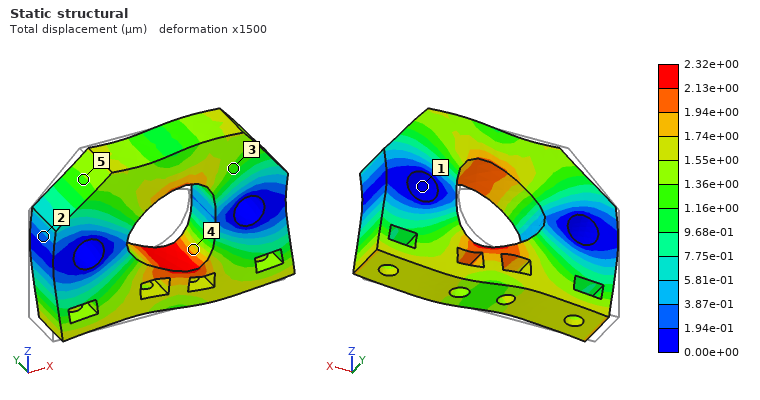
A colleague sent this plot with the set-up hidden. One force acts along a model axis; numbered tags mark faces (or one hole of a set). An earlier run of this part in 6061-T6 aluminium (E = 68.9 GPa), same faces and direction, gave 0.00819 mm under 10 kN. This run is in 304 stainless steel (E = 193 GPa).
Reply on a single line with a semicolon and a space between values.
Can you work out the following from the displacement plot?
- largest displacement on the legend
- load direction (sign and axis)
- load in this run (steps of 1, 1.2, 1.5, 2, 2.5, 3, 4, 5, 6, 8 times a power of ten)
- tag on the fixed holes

2.32e+00 µm; +X; 8 kN; 1
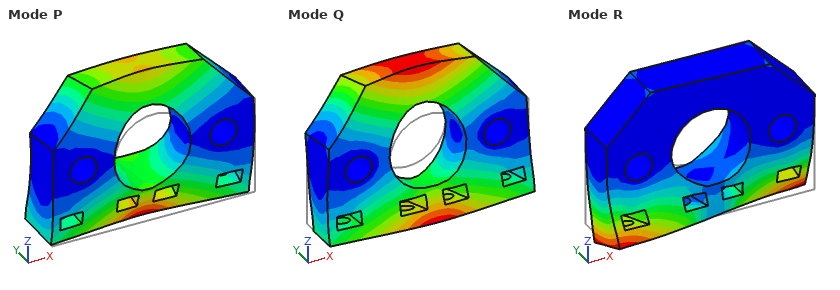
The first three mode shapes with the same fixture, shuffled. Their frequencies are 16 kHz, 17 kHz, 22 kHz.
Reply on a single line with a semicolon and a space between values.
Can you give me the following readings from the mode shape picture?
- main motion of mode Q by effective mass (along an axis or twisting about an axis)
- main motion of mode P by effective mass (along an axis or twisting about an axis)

twisting about X; along Y
